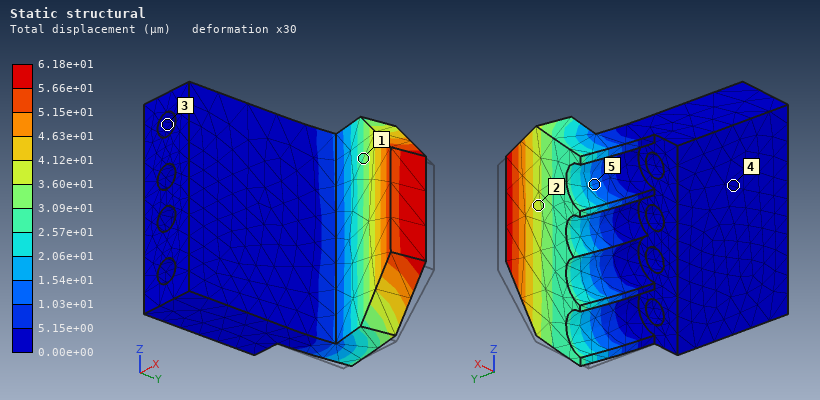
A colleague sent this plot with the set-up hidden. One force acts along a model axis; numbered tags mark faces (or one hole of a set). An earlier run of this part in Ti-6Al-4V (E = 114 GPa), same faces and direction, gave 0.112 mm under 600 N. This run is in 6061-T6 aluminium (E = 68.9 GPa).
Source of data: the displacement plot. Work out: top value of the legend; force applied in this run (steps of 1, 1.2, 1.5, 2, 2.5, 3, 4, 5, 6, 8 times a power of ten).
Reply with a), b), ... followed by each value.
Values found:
a) 6.18e+01 µm
b) 200 N
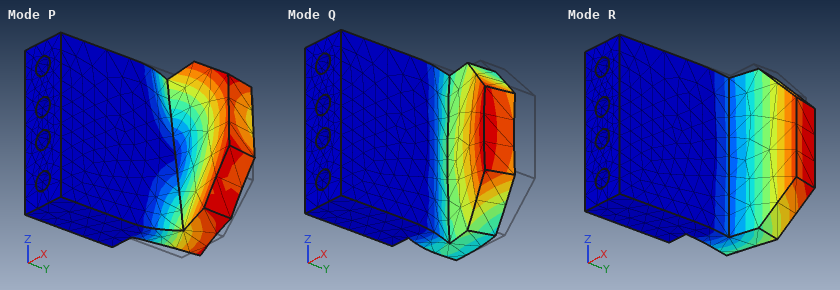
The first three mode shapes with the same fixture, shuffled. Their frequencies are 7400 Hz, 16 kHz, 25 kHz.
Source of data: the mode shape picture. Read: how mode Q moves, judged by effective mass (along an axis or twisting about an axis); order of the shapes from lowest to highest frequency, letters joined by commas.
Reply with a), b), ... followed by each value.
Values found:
a) along X
b) R, P, Q
